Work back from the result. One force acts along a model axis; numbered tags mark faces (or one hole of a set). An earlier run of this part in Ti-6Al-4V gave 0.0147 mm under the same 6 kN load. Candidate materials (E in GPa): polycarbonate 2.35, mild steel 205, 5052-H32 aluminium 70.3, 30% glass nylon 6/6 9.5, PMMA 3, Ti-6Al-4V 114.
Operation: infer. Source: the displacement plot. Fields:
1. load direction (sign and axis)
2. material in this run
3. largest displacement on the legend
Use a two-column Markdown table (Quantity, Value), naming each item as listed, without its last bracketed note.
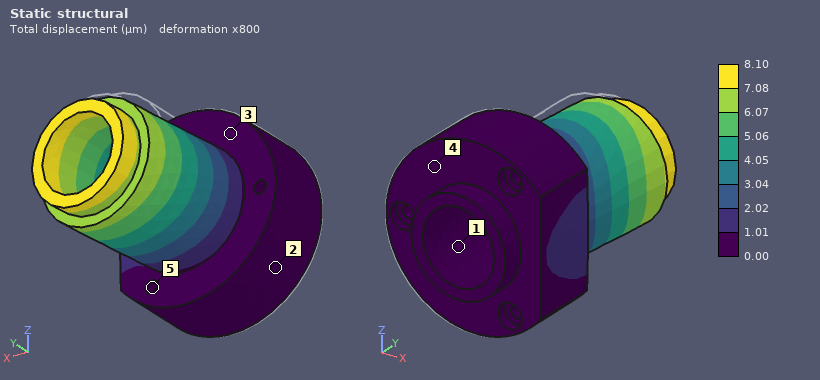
| Quantity | Value |
|---|---|
| load direction | +X |
| material in this run | mild steel |
| largest displacement on the legend | 8.10 µm |
